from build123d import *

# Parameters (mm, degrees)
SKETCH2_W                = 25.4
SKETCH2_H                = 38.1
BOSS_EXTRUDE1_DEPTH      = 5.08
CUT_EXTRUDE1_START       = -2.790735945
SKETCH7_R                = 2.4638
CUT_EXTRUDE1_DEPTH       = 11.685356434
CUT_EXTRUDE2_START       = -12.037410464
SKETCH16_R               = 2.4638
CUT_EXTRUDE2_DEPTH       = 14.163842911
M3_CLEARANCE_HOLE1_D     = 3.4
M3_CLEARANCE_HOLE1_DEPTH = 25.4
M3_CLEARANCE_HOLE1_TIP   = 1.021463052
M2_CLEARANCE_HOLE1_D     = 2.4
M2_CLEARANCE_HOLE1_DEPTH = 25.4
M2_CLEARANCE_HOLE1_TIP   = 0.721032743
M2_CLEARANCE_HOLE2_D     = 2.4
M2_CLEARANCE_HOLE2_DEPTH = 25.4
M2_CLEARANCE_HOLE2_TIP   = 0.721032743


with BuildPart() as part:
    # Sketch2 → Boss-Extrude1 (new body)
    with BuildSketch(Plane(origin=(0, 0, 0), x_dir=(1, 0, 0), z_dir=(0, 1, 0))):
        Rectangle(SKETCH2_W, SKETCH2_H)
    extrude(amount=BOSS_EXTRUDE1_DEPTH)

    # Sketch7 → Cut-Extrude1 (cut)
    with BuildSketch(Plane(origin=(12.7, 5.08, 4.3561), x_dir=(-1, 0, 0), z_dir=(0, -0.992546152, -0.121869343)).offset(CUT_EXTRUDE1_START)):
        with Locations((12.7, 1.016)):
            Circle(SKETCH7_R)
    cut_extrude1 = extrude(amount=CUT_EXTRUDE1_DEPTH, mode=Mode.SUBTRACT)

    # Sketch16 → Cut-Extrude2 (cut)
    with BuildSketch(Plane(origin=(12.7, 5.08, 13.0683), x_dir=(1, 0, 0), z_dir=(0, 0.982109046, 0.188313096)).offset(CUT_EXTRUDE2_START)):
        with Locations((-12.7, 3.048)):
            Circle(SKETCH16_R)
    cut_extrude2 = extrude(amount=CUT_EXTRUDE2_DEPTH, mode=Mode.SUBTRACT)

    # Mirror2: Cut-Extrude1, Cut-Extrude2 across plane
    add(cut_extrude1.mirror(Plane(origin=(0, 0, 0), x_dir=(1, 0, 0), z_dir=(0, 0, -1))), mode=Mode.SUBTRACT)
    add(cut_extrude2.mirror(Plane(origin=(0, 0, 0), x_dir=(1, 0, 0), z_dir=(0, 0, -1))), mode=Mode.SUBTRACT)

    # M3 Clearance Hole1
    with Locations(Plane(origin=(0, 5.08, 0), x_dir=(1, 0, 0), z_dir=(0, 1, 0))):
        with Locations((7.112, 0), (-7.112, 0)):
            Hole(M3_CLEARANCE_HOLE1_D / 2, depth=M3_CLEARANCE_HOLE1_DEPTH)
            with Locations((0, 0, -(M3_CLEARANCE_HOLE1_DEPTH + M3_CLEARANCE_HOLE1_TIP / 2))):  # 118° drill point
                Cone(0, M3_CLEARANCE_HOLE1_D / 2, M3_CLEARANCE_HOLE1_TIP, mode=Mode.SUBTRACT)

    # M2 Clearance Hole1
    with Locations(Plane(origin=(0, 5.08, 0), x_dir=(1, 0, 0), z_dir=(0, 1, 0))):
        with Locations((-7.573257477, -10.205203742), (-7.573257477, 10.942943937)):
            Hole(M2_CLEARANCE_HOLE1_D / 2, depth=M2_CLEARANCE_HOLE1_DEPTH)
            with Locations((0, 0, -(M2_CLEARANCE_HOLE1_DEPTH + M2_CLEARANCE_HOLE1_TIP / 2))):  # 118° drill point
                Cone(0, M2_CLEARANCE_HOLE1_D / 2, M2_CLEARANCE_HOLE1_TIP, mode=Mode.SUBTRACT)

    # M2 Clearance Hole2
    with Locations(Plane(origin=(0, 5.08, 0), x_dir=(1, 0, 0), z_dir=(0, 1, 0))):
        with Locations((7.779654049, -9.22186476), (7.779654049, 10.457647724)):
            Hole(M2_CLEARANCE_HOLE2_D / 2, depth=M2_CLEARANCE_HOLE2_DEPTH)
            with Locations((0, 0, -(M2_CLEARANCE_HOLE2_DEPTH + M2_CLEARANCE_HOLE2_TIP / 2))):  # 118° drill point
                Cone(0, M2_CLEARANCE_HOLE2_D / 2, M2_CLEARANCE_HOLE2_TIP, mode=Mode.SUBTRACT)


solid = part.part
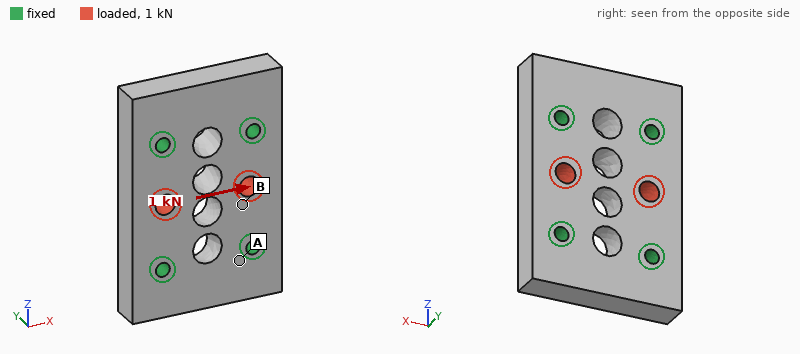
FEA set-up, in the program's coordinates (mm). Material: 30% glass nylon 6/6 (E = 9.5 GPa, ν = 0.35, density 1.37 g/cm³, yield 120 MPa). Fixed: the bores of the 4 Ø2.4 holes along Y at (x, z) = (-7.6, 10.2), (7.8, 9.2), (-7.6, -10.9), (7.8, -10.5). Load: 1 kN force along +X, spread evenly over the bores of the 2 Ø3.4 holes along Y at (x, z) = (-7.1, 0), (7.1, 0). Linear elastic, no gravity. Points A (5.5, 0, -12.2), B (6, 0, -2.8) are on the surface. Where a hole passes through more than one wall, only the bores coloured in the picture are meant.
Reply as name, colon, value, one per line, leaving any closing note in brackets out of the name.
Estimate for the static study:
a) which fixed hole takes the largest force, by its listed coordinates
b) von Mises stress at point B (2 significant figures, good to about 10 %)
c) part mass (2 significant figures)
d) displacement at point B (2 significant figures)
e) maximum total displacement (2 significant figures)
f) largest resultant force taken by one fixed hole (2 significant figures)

which fixed hole takes the largest force, by its listed coordinates: (7.8, 9.2)
von Mises stress at point B: 9.9 MPa
part mass: 5.9 g
displacement at point B: 15 µm
maximum total displacement: 21 µm
largest resultant force taken by one fixed hole: 300 N
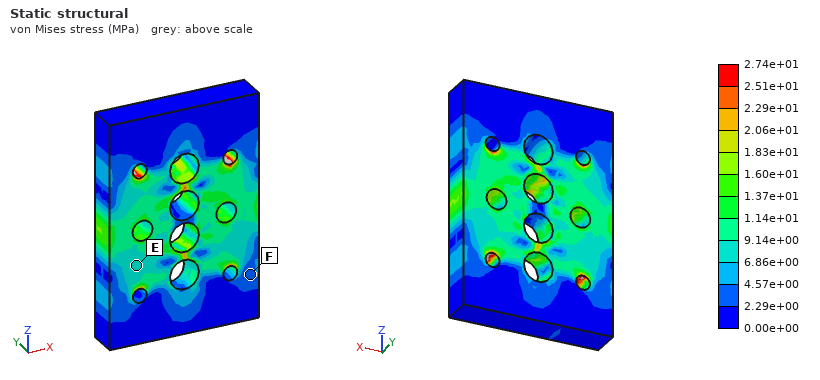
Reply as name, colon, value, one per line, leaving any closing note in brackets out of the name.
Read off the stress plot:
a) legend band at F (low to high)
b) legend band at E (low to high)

legend band at F: 2.29e+00 to 4.57e+00 MPa
legend band at E: 6.86e+00 to 9.14e+00 MPa
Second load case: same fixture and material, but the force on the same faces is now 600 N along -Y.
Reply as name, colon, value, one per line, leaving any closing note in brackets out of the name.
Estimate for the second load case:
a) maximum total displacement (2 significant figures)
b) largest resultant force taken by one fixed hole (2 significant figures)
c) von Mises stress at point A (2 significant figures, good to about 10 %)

maximum total displacement: 28 µm
largest resultant force taken by one fixed hole: 170 N
von Mises stress at point A: 4.5 MPa
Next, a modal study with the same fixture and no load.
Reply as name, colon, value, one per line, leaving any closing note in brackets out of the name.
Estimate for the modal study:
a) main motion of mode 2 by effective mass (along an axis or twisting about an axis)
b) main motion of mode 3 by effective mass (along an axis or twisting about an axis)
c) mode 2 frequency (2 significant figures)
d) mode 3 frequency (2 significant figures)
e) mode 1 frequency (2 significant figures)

main motion of mode 2 by effective mass: twisting about X
main motion of mode 3 by effective mass: along Y
mode 2 frequency: 20 kHz
mode 3 frequency: 23 kHz
mode 1 frequency: 17 kHz
